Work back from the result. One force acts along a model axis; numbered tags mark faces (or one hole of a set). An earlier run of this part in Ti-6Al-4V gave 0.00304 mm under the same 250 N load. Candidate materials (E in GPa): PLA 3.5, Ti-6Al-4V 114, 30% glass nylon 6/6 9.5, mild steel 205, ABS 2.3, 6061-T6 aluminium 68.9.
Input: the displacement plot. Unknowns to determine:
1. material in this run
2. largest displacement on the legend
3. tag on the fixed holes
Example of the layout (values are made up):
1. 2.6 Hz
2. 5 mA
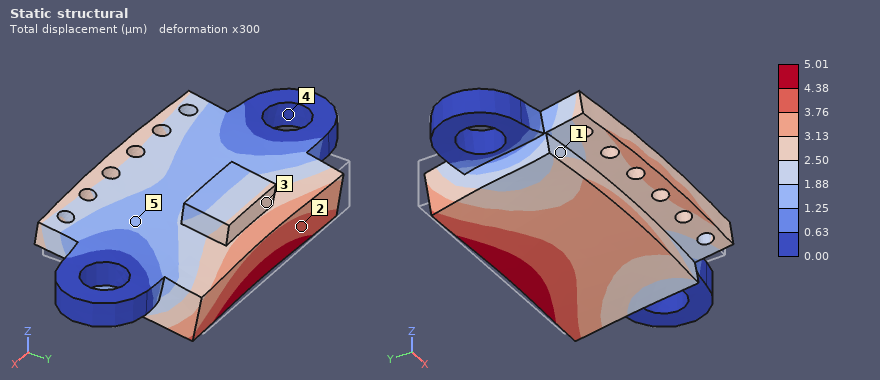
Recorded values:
1. 6061-T6 aluminium
2. 5.01 µm
3. 4
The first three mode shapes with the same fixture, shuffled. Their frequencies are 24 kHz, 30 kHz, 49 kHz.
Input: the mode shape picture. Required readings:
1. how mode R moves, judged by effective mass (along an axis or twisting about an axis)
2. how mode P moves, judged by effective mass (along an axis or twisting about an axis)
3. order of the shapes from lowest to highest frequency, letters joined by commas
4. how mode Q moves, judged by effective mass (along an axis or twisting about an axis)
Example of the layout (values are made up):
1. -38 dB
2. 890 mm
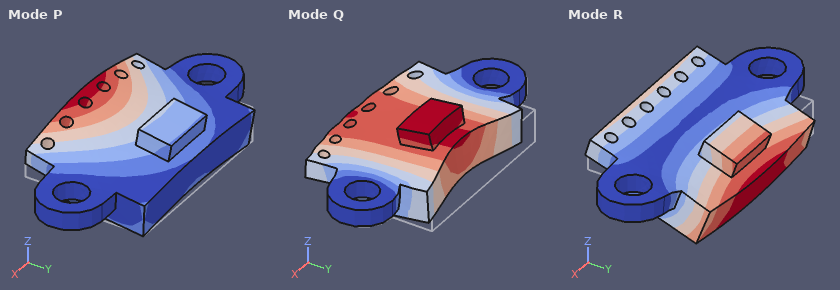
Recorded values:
1. along Z
2. along Z
3. R, P, Q
4. along Y
